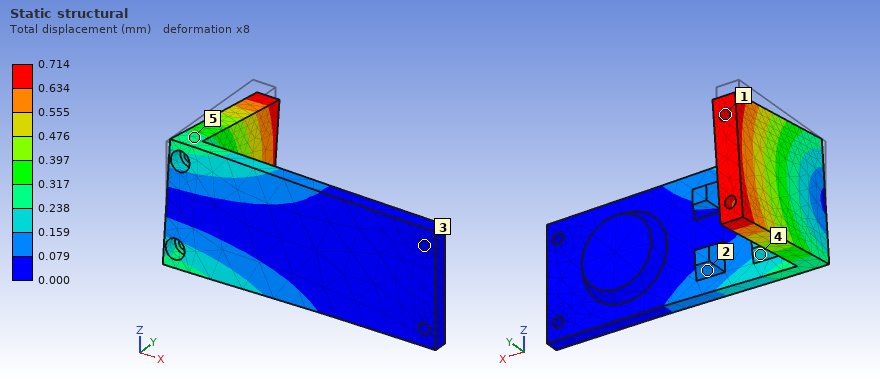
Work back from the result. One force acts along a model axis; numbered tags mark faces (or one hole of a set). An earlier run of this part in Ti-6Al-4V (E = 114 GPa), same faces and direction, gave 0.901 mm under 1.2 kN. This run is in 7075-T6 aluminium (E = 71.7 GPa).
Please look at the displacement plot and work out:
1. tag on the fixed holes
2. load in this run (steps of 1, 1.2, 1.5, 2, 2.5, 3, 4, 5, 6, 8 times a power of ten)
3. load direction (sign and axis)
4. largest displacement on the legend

3
600 N
-Z
0.714 mm
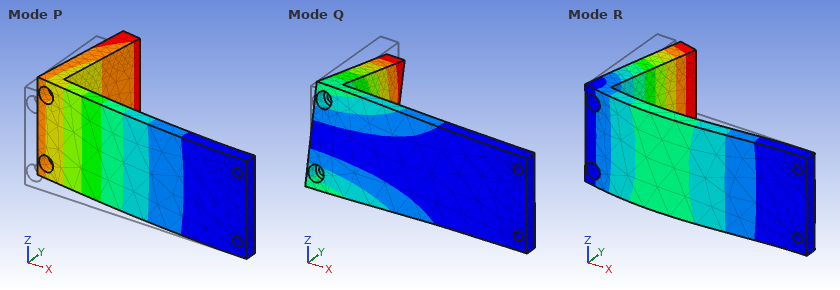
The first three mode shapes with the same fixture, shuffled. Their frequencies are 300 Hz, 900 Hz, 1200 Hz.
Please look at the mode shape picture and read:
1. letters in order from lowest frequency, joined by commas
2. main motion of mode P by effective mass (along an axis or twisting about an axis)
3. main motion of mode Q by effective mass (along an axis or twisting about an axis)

P, Q, R
along Y
along Z
